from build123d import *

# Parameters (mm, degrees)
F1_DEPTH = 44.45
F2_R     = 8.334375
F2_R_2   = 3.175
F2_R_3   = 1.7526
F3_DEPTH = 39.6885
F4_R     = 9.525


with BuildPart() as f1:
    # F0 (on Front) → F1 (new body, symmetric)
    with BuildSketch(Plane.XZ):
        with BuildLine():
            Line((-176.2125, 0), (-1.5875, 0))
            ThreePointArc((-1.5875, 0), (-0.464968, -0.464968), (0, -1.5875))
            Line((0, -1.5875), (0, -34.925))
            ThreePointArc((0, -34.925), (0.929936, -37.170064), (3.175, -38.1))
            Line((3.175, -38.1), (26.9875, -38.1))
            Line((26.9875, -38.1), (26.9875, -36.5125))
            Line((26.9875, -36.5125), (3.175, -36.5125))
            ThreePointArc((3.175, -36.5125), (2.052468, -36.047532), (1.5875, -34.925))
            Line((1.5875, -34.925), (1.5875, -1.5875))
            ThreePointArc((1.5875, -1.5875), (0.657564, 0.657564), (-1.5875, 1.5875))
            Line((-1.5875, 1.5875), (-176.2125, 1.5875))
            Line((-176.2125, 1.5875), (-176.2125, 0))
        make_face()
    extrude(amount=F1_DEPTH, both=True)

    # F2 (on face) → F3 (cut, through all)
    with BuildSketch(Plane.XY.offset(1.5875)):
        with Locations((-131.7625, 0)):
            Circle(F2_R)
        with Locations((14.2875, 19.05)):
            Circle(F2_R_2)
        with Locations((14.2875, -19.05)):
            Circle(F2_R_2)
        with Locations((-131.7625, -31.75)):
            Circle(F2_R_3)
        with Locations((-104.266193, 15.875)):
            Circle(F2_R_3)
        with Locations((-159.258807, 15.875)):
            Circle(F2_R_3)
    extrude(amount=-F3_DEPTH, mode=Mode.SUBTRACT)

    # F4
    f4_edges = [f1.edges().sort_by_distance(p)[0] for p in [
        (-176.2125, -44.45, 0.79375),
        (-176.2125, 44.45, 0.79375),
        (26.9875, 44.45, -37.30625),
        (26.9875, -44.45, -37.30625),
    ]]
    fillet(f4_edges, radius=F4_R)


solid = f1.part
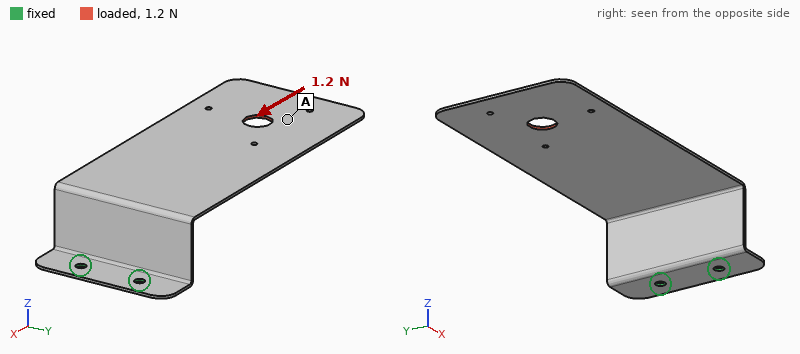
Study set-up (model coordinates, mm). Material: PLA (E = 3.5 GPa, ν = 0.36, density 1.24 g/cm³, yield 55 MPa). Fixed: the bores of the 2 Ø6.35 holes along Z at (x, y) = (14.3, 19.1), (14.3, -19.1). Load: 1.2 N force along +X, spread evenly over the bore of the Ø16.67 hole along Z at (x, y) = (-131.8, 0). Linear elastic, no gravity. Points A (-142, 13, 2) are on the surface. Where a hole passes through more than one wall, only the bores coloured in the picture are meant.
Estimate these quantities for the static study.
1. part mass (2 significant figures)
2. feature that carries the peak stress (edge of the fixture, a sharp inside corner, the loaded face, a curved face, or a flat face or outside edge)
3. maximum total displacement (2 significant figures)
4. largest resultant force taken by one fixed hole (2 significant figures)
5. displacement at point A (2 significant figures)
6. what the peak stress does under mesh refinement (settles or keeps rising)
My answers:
41 g
edge of the fixture
2.3 mm
0.60 N
1.9 mm
keeps rising
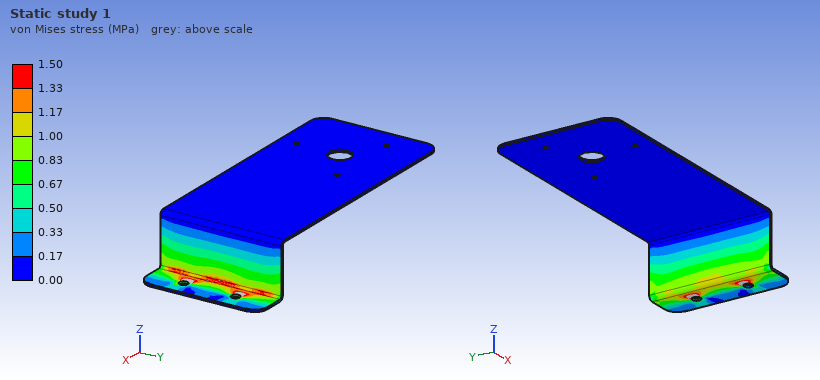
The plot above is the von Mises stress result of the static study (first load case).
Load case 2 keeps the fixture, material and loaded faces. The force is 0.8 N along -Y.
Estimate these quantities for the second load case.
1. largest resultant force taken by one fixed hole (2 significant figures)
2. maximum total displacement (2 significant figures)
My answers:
2.7 N
2.2 mm
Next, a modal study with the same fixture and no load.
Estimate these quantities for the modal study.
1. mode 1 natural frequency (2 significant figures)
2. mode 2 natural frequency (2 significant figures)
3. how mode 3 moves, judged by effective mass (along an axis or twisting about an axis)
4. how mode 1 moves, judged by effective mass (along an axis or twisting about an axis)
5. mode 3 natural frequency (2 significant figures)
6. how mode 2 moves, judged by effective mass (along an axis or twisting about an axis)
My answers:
9.8 Hz
26 Hz
along X
along Z
54 Hz
along Y
